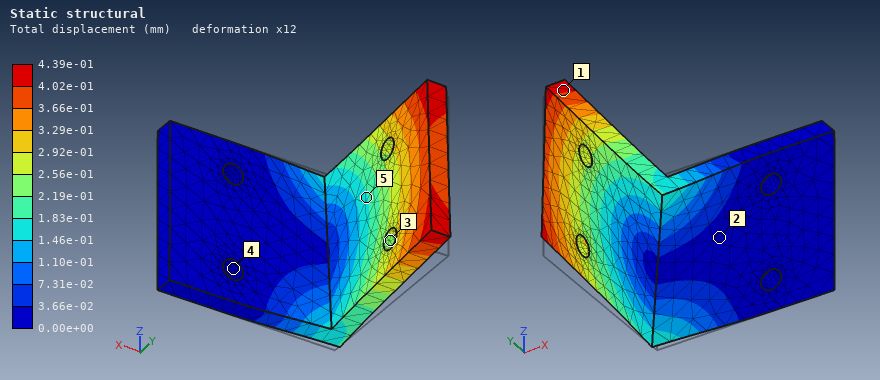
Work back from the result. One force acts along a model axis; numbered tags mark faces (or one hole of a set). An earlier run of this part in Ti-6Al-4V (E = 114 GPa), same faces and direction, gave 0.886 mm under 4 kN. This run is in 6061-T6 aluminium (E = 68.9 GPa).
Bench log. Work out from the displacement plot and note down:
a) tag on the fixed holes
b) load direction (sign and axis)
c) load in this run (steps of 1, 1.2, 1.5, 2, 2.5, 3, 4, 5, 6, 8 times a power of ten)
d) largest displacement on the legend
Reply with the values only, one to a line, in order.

4
+Z
1.2 kN
4.39e-01 mm
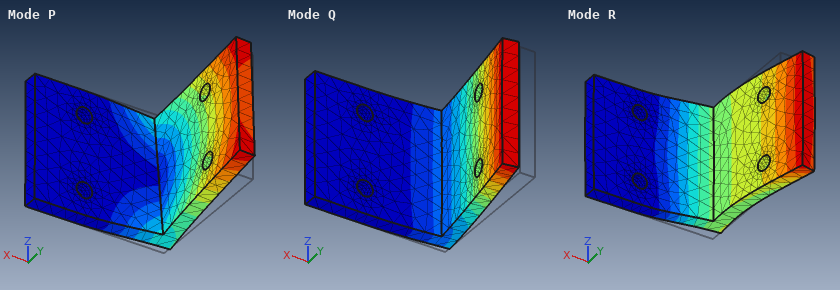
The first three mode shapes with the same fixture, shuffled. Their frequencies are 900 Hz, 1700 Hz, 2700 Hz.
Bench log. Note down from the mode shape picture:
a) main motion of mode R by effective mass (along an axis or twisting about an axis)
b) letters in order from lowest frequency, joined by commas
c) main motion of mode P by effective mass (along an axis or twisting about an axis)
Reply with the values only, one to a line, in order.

along Y
Q, P, R
along Z
